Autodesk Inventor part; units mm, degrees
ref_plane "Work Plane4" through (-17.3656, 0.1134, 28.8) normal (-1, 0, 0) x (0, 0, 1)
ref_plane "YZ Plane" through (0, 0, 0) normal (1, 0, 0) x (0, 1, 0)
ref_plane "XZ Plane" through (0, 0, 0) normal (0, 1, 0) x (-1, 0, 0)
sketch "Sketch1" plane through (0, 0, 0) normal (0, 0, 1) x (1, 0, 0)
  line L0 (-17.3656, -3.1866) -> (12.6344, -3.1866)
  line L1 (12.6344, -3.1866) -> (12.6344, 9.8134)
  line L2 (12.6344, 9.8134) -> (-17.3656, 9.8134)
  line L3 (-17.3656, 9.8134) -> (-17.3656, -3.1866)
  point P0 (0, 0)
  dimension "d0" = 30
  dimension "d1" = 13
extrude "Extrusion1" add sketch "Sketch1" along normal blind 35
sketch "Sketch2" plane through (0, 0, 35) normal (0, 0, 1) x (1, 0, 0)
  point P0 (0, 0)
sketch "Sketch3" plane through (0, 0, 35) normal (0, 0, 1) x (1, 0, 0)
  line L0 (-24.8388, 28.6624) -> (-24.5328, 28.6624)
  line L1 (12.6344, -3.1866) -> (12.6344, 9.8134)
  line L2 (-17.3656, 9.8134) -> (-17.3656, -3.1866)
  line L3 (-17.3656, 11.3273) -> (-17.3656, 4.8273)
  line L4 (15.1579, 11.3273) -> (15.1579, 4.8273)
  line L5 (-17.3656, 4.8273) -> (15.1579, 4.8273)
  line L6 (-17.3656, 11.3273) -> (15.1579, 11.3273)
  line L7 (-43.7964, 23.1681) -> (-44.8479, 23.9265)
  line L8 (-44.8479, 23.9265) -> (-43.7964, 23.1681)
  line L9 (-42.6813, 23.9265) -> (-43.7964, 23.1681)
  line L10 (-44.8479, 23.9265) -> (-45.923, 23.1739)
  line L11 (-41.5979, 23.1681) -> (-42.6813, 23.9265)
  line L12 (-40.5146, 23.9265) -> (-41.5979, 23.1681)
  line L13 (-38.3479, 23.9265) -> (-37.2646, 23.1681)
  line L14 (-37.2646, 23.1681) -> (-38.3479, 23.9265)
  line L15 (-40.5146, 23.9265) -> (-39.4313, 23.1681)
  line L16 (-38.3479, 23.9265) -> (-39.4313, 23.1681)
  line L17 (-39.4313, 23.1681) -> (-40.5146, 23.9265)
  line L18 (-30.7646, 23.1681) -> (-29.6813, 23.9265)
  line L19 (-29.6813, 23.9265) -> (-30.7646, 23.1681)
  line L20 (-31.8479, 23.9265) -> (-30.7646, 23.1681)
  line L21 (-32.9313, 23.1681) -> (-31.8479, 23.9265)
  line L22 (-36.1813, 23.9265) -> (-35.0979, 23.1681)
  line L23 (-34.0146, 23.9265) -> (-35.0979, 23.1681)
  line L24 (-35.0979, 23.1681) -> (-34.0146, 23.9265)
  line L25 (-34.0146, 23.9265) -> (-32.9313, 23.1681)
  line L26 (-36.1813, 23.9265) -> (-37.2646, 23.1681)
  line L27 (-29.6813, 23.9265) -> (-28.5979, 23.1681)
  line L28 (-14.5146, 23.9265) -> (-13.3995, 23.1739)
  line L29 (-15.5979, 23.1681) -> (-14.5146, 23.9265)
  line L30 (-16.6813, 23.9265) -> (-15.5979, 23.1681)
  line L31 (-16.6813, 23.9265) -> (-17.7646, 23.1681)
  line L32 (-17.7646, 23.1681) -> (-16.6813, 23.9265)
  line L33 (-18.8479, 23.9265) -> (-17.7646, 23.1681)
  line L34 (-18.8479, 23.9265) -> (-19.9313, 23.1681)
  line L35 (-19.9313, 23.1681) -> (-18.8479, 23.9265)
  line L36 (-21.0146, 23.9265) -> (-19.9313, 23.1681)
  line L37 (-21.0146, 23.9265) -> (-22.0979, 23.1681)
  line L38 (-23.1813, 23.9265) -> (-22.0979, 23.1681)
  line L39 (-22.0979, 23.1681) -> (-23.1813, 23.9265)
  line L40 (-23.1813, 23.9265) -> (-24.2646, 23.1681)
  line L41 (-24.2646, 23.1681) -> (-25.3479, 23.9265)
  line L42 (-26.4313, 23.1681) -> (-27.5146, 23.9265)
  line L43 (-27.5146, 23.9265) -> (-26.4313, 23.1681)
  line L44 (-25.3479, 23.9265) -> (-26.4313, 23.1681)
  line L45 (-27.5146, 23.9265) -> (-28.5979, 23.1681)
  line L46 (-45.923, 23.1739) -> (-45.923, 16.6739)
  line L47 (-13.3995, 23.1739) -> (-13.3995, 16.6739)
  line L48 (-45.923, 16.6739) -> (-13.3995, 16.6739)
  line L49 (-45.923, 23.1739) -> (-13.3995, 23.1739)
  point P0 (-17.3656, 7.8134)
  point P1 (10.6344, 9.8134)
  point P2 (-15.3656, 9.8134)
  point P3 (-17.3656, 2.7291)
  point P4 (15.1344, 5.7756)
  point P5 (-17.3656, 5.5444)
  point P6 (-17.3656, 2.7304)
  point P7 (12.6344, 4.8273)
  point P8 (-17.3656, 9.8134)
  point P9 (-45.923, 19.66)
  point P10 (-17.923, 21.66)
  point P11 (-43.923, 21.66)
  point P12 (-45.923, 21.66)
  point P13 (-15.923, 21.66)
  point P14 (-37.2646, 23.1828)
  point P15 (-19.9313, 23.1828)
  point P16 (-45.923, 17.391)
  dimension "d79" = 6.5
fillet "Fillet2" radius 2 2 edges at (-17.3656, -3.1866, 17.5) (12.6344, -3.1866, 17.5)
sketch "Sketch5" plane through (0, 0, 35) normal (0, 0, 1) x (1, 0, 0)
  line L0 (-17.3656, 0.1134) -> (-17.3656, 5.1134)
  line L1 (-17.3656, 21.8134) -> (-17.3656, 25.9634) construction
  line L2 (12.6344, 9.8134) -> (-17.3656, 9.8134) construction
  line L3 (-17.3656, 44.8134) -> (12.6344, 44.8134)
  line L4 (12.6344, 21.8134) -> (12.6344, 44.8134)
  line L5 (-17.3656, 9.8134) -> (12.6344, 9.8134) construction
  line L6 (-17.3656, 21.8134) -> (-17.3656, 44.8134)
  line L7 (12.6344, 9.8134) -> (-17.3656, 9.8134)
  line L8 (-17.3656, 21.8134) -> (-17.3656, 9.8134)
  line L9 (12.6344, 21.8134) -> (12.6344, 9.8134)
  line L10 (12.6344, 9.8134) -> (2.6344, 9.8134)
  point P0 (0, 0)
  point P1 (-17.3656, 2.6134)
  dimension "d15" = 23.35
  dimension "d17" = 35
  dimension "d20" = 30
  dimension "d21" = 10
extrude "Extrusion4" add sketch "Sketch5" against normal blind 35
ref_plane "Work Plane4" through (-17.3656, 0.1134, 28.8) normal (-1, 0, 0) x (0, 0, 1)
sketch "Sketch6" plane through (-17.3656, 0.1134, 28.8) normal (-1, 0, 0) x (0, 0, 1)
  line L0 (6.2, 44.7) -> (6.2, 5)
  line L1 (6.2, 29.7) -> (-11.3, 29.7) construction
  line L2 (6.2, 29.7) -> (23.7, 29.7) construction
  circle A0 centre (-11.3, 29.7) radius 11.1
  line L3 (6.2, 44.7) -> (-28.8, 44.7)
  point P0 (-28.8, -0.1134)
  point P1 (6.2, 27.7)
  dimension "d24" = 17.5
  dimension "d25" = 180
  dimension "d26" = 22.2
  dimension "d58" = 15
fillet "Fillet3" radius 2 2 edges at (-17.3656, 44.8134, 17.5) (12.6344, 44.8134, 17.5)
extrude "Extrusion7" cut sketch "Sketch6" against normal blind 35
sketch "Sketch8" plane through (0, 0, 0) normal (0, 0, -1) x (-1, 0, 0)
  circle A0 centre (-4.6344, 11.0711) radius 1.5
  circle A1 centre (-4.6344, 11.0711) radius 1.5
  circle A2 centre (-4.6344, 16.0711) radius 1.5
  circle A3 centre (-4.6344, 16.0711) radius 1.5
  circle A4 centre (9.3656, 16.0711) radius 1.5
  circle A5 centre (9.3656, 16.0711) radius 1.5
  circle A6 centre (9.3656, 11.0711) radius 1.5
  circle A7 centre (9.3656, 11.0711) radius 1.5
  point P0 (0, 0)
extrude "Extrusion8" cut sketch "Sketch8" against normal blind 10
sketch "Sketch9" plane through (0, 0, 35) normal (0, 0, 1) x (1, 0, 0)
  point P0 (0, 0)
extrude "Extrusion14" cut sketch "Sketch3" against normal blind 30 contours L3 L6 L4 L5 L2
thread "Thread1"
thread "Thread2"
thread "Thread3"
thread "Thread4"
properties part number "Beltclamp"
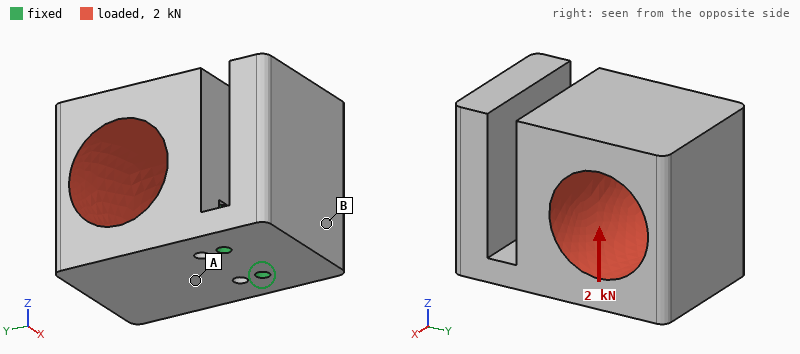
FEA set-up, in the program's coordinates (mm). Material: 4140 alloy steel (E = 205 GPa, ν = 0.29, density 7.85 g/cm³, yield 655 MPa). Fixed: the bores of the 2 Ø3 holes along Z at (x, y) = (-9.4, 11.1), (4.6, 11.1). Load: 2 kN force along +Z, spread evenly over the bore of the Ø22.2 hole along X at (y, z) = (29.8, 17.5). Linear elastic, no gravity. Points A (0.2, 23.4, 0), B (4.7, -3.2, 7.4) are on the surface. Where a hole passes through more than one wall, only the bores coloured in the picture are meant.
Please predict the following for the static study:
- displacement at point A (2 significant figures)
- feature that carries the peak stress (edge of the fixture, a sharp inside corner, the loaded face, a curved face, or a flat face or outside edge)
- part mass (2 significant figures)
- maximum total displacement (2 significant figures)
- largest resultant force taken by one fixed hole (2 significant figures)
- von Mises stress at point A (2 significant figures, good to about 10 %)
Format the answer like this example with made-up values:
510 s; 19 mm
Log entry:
8.5 µm; a flat face or outside edge; 260 g; 39 µm; 1.0 kN; 29 MPa
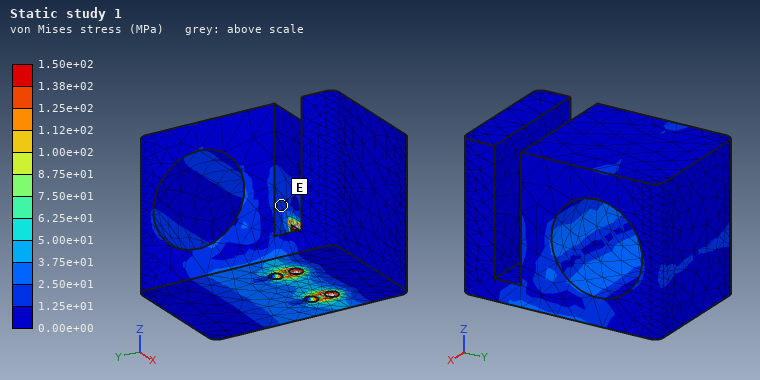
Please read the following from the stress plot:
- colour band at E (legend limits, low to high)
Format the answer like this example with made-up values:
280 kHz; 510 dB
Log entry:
1.25e+01 to 2.50e+01 MPa
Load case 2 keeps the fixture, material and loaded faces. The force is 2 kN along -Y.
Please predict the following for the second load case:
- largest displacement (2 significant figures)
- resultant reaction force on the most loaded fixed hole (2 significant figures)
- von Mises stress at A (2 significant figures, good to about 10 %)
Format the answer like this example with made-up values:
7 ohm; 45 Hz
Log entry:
29 µm; 1.0 kN; 12 MPa
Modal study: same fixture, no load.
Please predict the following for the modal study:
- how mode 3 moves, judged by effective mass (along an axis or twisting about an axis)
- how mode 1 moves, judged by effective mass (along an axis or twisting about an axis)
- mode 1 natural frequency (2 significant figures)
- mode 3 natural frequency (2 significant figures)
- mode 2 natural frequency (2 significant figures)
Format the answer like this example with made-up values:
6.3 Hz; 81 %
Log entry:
along X; along Y; 2600 Hz; 5500 Hz; 2900 Hz
